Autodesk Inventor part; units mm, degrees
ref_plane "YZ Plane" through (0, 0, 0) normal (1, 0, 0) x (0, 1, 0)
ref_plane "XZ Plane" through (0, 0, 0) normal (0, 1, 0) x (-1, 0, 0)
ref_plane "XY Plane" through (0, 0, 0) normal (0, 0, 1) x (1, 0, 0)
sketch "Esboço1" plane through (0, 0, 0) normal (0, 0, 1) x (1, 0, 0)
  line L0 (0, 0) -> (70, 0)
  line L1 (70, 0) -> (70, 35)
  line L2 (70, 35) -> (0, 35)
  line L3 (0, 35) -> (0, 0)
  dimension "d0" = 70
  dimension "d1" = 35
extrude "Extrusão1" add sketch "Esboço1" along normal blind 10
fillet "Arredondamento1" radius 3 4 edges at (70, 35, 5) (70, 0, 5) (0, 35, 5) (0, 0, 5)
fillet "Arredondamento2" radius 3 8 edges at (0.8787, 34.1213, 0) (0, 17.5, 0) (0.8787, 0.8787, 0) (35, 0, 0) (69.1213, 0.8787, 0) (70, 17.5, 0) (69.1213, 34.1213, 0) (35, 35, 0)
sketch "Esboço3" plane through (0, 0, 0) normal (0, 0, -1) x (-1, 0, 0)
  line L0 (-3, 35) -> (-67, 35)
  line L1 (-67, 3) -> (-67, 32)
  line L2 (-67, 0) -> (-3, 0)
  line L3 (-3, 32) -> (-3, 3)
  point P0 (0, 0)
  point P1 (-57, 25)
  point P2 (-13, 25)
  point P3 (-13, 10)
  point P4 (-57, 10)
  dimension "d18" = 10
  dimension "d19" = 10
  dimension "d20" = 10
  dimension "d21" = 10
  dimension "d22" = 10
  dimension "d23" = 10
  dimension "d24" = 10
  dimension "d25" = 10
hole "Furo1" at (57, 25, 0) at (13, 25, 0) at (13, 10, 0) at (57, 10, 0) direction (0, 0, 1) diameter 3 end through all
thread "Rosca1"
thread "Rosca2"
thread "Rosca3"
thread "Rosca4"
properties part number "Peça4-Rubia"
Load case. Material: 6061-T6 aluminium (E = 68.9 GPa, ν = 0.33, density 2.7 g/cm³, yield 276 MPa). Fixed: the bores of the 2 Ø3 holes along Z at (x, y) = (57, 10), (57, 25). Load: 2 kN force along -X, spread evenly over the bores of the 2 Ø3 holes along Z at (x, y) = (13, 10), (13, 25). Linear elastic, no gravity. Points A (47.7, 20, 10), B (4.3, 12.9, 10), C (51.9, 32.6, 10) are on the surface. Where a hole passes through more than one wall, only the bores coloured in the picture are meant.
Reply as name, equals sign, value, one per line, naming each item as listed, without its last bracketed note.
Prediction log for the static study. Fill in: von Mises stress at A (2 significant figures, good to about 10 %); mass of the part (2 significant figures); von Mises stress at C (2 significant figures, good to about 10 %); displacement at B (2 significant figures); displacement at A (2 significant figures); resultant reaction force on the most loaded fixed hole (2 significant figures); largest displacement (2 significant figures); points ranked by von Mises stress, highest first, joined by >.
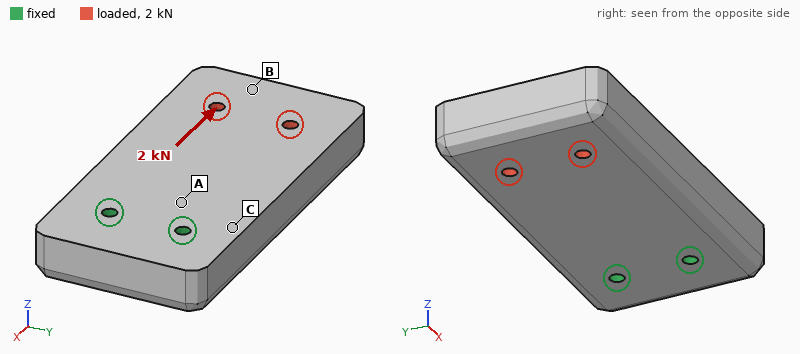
von Mises stress at A = 6.1 MPa
mass of the part = 64 g
von Mises stress at C = 3.3 MPa
displacement at B = 4.3 µm
displacement at A = 1.0 µm
resultant reaction force on the most loaded fixed hole = 1.0 kN
largest displacement = 4.8 µm
points ranked by von Mises stress, highest first, joined by > = A > C > B
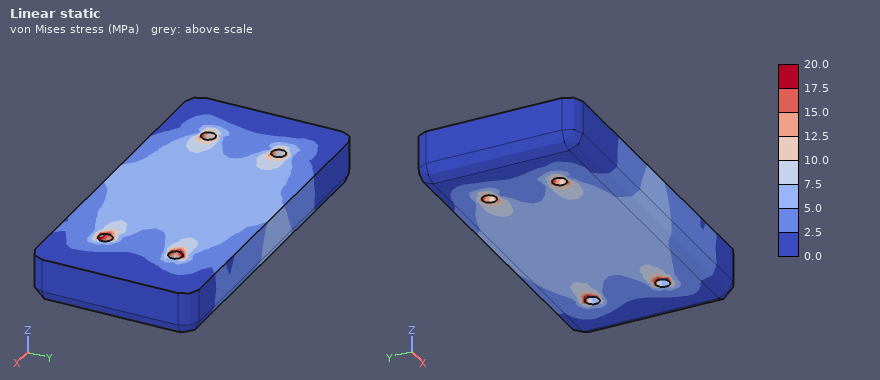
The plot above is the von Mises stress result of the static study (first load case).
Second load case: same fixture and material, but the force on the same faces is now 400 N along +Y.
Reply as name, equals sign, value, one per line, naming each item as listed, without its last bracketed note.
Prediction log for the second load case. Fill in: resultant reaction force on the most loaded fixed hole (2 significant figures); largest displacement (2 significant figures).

resultant reaction force on the most loaded fixed hole = 1.1 kN
largest displacement = 15 µm
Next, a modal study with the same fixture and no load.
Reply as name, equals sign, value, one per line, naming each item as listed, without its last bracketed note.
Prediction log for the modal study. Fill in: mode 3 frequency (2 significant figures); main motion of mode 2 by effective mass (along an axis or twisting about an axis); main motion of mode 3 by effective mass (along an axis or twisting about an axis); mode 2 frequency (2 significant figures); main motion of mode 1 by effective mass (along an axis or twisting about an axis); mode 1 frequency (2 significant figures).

mode 3 frequency = 7400 Hz
main motion of mode 2 by effective mass = along Y
main motion of mode 3 by effective mass = twisting about X
mode 2 frequency = 5600 Hz
main motion of mode 1 by effective mass = along Z
mode 1 frequency = 2300 Hz
